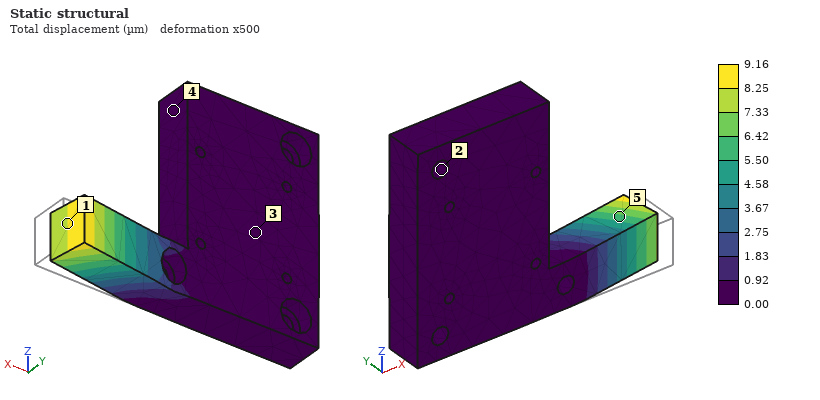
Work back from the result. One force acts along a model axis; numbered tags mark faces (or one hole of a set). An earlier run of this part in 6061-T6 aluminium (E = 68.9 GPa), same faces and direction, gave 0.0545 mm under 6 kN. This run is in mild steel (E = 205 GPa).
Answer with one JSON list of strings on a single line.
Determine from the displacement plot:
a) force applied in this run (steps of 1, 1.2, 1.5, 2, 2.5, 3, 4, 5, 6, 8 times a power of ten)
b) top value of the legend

["3 kN", "9.16 µm"]
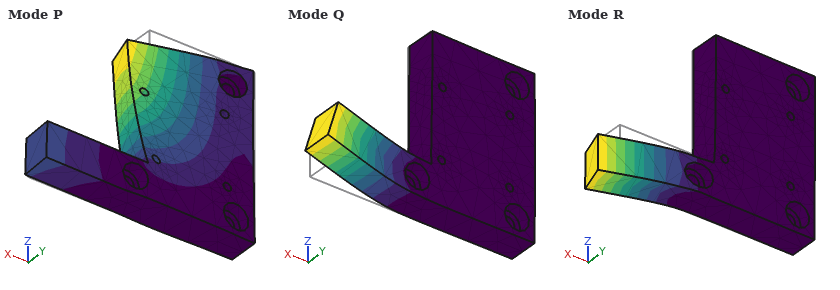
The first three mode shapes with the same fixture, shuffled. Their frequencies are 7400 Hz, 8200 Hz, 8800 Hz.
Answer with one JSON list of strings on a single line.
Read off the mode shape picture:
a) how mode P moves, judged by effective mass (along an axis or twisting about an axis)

["along Y"]
